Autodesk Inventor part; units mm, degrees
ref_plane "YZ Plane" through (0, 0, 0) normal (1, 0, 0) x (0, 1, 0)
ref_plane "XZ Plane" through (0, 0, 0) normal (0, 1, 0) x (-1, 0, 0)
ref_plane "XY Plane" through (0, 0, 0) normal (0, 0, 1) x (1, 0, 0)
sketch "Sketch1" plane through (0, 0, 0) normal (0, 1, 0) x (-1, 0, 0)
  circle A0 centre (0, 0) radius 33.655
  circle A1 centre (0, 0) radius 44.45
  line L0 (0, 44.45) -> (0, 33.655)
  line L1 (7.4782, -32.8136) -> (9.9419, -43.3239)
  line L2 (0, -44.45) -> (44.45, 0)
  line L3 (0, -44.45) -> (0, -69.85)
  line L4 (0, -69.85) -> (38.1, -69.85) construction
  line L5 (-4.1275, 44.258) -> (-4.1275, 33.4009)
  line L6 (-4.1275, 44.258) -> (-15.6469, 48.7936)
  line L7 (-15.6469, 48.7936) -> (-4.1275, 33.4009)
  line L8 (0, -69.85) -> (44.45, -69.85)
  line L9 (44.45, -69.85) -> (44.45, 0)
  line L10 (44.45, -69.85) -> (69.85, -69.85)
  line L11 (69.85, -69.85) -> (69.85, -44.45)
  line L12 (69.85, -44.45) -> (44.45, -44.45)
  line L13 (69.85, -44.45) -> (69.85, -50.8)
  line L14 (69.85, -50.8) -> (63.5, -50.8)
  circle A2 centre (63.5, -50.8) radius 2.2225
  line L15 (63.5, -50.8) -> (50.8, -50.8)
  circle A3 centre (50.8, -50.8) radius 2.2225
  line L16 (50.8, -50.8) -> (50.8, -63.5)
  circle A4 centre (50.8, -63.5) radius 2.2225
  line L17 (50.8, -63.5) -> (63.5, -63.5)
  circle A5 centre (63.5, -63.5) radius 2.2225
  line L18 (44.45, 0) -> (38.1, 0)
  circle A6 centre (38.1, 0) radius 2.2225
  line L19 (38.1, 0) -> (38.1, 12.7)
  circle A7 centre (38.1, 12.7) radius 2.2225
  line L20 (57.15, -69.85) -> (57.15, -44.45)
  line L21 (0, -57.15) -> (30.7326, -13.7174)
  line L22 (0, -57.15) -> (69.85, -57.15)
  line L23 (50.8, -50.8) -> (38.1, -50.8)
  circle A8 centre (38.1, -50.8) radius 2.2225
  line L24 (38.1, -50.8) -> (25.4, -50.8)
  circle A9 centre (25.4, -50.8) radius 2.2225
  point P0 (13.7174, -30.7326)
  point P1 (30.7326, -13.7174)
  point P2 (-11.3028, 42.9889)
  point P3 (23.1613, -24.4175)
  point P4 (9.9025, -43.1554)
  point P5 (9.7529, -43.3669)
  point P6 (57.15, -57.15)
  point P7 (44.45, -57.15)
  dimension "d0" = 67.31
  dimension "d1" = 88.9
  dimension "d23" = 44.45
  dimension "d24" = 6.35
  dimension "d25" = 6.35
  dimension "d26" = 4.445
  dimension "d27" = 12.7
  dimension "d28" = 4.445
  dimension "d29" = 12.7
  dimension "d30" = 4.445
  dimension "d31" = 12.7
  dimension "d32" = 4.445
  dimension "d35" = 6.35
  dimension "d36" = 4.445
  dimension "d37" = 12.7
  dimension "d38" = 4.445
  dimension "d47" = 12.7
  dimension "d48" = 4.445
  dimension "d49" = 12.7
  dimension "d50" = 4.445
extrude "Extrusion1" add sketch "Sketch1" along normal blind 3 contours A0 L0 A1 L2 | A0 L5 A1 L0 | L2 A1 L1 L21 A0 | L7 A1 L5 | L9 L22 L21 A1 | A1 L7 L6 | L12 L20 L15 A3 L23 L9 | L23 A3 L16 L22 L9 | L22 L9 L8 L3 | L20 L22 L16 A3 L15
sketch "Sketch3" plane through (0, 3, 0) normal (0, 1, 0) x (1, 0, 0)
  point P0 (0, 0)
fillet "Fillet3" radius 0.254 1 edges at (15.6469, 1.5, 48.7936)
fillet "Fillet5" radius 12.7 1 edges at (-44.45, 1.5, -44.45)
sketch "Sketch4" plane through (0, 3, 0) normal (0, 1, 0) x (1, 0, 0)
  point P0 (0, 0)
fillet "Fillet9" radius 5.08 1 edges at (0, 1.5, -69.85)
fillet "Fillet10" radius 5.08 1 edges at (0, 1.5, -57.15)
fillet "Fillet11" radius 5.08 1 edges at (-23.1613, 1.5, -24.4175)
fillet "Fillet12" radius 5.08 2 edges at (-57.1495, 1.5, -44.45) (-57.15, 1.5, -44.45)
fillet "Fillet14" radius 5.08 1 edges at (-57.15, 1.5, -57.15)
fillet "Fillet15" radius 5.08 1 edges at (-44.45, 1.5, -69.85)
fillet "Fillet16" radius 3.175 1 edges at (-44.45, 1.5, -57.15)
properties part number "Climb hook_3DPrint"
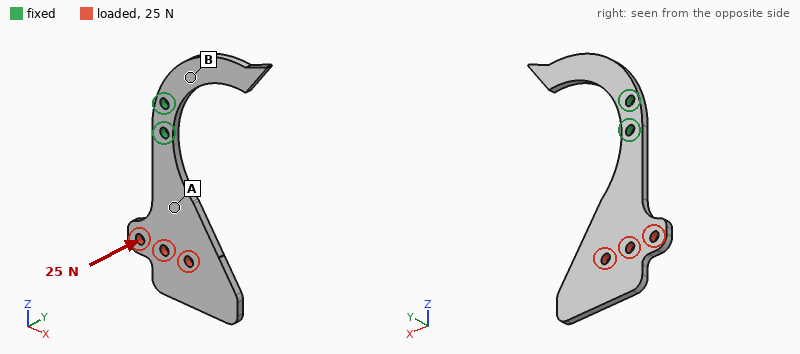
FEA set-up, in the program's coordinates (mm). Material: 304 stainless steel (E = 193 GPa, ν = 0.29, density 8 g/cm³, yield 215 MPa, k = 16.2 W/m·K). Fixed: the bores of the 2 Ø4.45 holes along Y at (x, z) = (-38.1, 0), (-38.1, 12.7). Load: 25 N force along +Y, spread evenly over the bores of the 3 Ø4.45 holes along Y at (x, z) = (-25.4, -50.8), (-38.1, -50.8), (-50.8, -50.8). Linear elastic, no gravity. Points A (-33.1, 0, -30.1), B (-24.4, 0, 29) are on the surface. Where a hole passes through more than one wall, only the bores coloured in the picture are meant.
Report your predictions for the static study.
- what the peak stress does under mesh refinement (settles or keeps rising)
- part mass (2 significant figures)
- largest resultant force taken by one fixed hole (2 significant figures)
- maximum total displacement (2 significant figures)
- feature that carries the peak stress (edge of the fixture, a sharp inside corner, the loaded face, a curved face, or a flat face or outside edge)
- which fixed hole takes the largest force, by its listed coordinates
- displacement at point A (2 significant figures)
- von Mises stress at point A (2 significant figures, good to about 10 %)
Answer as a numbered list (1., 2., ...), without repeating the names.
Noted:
1. keeps rising
2. 68 g
3. 30 N
4. 0.26 mm
5. edge of the fixture
6. (-38.1, 0)
7. 0.077 mm
8. 14 MPa
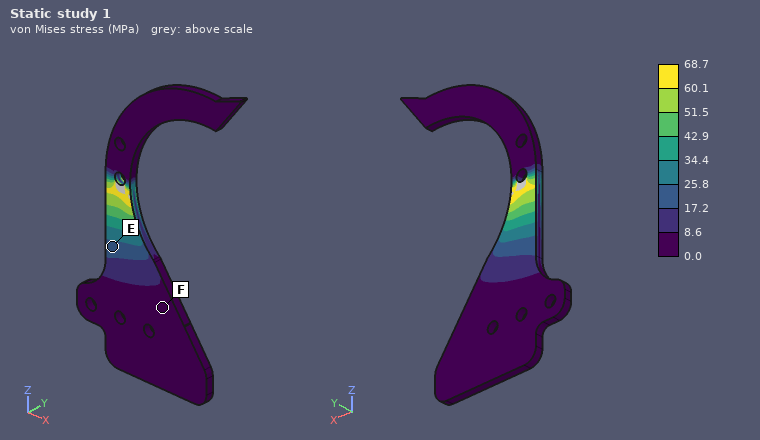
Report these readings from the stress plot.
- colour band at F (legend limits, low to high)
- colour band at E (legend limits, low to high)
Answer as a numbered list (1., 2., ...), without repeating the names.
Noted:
1. 0.0 to 8.6 MPa
2. 17.2 to 25.8 MPa
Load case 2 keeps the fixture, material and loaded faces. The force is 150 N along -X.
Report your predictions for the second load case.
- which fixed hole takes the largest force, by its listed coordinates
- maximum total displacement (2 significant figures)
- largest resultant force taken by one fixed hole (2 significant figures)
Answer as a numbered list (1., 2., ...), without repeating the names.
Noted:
1. (-38.1, 0)
2. 0.13 mm
3. 370 N
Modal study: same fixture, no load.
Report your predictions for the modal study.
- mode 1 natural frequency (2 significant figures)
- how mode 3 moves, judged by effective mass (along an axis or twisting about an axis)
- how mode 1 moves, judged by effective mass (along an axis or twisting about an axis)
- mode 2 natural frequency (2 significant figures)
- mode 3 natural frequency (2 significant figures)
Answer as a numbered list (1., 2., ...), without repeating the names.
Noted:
1. 280 Hz
2. twisting about Z
3. along Y
4. 750 Hz
5. 940 Hz
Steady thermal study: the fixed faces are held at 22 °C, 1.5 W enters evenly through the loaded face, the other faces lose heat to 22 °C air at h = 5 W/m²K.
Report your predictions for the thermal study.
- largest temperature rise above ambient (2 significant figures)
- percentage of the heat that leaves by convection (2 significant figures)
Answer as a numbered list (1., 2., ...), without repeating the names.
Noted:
1. 49 K
2. 55 %
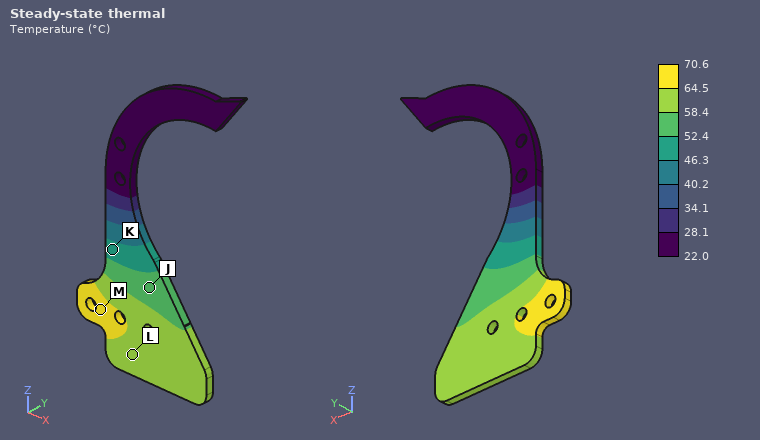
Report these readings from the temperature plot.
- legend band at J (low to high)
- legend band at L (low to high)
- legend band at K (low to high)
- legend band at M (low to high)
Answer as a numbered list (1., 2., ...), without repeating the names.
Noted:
1. 52.4 to 58.4 °C
2. 58.4 to 64.5 °C
3. 46.3 to 52.4 °C
4. 64.5 to 70.6 °C
